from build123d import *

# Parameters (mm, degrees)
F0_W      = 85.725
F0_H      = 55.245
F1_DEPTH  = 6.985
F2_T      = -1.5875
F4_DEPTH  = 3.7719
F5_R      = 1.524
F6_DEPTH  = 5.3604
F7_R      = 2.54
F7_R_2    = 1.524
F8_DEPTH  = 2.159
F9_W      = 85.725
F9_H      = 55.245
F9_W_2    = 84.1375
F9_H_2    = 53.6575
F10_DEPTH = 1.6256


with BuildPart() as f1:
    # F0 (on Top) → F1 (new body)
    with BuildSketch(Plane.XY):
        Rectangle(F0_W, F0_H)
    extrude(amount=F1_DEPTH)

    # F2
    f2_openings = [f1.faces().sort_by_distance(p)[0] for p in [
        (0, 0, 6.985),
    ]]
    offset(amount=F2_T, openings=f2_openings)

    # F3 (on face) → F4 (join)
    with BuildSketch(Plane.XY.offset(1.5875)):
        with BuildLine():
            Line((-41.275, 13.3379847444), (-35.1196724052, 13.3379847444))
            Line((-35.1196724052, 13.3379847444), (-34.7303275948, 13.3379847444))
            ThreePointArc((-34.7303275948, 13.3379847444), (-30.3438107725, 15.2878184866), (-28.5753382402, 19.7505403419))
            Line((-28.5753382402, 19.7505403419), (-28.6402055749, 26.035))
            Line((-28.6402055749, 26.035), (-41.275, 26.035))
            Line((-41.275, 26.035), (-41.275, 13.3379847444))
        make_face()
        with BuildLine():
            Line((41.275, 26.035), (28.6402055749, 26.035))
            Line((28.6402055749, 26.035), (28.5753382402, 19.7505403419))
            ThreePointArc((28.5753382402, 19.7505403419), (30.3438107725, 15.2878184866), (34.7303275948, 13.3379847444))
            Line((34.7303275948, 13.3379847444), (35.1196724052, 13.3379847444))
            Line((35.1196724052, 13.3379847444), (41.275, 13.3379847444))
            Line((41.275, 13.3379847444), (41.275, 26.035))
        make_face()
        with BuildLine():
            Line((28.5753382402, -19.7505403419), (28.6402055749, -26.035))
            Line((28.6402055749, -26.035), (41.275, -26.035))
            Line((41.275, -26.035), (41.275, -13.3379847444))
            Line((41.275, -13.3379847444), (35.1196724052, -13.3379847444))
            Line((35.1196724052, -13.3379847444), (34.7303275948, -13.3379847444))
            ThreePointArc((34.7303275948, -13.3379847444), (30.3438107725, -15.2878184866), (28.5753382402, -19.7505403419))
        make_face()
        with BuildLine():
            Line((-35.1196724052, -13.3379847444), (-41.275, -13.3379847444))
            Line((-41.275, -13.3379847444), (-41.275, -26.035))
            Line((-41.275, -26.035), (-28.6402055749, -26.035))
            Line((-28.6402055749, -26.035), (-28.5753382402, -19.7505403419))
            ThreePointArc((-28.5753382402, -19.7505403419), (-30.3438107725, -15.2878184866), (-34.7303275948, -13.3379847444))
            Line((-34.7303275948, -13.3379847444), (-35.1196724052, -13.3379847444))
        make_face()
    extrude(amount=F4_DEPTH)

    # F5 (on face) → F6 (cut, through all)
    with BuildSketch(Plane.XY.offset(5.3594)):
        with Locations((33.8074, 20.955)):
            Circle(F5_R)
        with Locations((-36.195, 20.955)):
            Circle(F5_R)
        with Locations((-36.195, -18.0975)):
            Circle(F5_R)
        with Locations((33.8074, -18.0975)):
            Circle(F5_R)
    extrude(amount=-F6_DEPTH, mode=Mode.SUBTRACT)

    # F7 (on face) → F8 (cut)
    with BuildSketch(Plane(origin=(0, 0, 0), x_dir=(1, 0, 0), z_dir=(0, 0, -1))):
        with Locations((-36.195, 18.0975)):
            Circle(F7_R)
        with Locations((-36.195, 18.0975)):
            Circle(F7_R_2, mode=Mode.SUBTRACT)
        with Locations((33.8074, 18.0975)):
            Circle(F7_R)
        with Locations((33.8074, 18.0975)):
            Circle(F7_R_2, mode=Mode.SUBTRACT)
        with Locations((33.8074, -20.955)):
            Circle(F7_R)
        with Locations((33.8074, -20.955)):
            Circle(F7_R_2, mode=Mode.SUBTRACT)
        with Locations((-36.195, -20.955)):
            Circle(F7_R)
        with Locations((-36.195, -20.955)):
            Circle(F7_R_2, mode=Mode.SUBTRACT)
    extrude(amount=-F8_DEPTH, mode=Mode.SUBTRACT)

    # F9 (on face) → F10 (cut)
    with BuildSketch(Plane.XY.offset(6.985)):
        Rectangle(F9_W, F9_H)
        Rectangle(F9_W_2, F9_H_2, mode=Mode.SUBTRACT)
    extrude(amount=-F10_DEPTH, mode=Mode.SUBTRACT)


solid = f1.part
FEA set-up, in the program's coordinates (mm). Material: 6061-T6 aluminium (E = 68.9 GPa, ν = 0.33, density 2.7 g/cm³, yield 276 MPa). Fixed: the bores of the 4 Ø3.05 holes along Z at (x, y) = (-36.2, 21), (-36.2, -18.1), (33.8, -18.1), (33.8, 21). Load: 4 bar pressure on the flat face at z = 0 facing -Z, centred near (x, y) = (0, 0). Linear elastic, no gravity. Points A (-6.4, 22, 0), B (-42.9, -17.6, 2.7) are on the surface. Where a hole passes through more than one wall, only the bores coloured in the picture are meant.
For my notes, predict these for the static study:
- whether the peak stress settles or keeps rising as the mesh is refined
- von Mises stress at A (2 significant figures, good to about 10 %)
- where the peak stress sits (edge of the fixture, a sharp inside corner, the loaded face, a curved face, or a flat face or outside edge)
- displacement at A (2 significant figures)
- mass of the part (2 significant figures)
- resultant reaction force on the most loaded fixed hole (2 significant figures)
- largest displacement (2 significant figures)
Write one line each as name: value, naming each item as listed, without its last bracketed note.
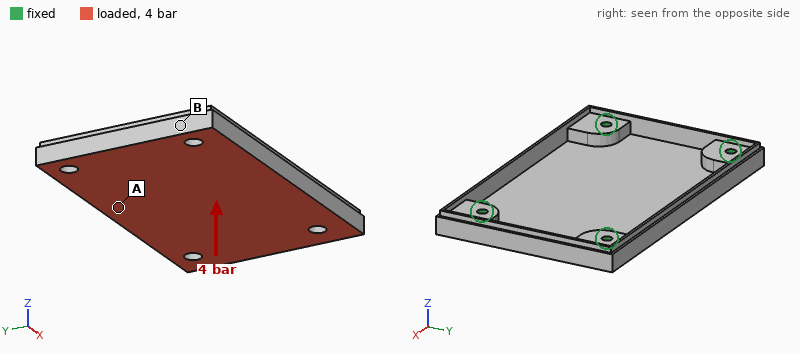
whether the peak stress settles or keeps rising as the mesh is refined: keeps rising
von Mises stress at A: 61 MPa
where the peak stress sits: edge of the fixture
displacement at A: 0.20 mm
mass of the part: 31 g
resultant reaction force on the most loaded fixed hole: 710 N
largest displacement: 0.50 mm
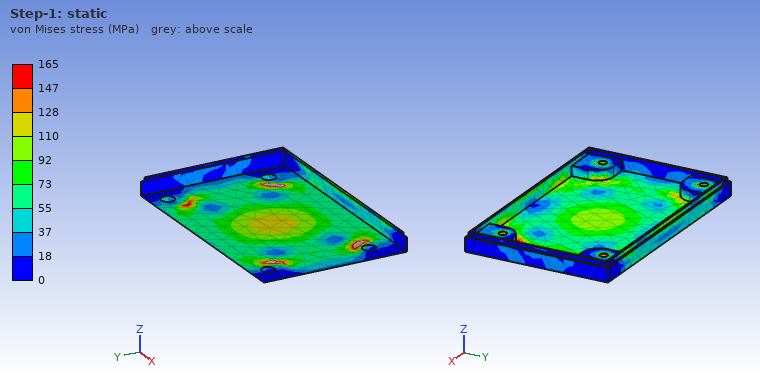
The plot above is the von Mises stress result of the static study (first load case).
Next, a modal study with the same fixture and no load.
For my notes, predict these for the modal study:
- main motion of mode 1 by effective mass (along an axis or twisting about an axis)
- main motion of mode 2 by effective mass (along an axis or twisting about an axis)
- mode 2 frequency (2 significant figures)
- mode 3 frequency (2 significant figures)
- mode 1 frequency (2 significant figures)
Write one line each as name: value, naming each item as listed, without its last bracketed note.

main motion of mode 1 by effective mass: along Z
main motion of mode 2 by effective mass: twisting about X
mode 2 frequency: 4900 Hz
mode 3 frequency: 5700 Hz
mode 1 frequency: 2700 Hz
